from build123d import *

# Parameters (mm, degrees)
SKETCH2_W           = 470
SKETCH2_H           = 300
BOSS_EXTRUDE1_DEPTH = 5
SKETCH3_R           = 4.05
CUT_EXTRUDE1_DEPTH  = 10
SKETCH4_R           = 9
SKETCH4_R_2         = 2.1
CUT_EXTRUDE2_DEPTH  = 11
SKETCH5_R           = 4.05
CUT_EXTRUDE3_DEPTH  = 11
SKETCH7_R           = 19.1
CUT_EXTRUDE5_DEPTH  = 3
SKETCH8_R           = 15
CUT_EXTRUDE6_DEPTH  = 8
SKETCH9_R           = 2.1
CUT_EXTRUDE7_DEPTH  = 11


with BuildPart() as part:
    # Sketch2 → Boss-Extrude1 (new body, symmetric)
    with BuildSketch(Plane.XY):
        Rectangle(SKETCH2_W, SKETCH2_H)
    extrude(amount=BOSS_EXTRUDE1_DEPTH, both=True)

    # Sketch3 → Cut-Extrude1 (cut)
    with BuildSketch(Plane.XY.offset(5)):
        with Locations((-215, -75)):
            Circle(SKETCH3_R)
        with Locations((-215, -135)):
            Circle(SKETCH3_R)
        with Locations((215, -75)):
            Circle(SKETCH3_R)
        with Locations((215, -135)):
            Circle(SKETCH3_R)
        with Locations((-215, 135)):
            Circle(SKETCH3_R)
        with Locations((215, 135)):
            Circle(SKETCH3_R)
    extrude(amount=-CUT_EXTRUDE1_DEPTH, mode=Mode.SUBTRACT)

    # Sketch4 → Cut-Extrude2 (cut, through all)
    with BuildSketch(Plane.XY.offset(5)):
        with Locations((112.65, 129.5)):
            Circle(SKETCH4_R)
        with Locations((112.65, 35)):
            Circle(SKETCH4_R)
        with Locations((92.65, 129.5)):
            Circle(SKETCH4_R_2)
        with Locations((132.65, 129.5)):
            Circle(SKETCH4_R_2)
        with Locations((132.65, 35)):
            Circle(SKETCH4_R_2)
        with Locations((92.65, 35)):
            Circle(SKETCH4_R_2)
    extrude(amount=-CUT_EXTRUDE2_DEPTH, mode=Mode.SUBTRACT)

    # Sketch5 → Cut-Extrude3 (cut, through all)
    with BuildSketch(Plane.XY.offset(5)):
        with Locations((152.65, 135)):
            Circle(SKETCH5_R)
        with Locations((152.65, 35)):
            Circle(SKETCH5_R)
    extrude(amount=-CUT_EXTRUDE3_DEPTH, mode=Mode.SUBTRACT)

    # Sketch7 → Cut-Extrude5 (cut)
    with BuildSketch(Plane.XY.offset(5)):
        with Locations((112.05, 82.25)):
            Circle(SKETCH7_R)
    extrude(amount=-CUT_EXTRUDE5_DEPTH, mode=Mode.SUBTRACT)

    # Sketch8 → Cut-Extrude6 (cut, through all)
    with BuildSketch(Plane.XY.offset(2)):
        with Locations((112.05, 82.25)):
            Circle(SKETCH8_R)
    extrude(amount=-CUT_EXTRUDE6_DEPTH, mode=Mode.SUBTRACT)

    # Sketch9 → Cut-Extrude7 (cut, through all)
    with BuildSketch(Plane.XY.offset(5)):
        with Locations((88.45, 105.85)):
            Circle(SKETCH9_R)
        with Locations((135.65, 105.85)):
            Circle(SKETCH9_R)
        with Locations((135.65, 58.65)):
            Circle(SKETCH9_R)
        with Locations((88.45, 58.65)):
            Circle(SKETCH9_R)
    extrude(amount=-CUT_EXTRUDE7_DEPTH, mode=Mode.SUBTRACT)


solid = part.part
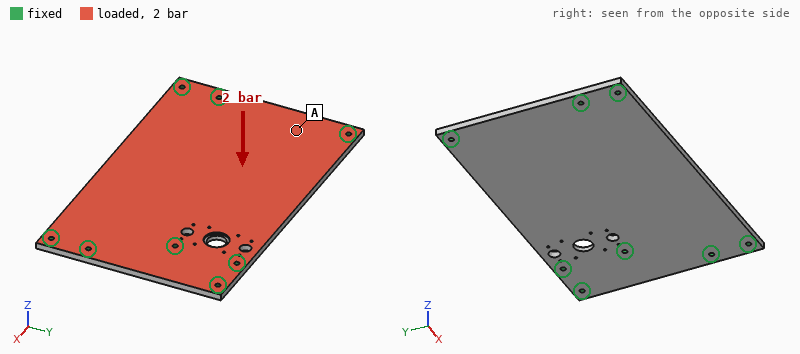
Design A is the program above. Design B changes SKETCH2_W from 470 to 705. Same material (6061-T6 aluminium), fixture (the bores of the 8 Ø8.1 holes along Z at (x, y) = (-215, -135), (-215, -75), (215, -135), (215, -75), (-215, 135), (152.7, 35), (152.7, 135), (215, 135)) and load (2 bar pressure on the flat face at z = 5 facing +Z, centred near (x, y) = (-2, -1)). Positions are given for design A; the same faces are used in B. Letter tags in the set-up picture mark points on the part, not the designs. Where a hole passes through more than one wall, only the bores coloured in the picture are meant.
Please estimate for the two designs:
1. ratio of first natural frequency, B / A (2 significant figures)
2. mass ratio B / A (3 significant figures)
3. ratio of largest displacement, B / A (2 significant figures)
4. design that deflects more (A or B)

0.97
1.51
0.88
A
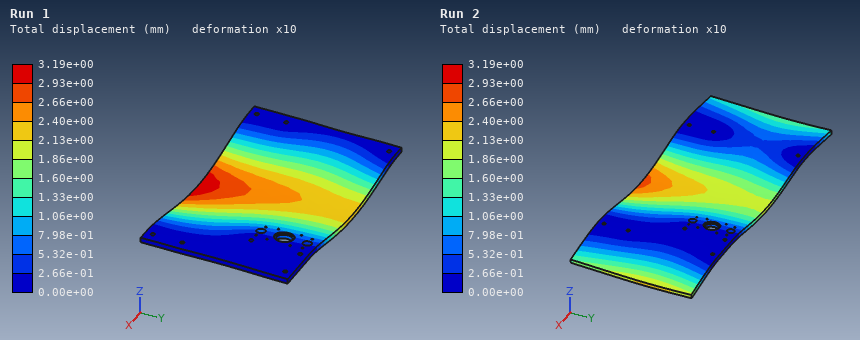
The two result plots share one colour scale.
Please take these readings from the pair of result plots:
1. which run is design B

Run 2
